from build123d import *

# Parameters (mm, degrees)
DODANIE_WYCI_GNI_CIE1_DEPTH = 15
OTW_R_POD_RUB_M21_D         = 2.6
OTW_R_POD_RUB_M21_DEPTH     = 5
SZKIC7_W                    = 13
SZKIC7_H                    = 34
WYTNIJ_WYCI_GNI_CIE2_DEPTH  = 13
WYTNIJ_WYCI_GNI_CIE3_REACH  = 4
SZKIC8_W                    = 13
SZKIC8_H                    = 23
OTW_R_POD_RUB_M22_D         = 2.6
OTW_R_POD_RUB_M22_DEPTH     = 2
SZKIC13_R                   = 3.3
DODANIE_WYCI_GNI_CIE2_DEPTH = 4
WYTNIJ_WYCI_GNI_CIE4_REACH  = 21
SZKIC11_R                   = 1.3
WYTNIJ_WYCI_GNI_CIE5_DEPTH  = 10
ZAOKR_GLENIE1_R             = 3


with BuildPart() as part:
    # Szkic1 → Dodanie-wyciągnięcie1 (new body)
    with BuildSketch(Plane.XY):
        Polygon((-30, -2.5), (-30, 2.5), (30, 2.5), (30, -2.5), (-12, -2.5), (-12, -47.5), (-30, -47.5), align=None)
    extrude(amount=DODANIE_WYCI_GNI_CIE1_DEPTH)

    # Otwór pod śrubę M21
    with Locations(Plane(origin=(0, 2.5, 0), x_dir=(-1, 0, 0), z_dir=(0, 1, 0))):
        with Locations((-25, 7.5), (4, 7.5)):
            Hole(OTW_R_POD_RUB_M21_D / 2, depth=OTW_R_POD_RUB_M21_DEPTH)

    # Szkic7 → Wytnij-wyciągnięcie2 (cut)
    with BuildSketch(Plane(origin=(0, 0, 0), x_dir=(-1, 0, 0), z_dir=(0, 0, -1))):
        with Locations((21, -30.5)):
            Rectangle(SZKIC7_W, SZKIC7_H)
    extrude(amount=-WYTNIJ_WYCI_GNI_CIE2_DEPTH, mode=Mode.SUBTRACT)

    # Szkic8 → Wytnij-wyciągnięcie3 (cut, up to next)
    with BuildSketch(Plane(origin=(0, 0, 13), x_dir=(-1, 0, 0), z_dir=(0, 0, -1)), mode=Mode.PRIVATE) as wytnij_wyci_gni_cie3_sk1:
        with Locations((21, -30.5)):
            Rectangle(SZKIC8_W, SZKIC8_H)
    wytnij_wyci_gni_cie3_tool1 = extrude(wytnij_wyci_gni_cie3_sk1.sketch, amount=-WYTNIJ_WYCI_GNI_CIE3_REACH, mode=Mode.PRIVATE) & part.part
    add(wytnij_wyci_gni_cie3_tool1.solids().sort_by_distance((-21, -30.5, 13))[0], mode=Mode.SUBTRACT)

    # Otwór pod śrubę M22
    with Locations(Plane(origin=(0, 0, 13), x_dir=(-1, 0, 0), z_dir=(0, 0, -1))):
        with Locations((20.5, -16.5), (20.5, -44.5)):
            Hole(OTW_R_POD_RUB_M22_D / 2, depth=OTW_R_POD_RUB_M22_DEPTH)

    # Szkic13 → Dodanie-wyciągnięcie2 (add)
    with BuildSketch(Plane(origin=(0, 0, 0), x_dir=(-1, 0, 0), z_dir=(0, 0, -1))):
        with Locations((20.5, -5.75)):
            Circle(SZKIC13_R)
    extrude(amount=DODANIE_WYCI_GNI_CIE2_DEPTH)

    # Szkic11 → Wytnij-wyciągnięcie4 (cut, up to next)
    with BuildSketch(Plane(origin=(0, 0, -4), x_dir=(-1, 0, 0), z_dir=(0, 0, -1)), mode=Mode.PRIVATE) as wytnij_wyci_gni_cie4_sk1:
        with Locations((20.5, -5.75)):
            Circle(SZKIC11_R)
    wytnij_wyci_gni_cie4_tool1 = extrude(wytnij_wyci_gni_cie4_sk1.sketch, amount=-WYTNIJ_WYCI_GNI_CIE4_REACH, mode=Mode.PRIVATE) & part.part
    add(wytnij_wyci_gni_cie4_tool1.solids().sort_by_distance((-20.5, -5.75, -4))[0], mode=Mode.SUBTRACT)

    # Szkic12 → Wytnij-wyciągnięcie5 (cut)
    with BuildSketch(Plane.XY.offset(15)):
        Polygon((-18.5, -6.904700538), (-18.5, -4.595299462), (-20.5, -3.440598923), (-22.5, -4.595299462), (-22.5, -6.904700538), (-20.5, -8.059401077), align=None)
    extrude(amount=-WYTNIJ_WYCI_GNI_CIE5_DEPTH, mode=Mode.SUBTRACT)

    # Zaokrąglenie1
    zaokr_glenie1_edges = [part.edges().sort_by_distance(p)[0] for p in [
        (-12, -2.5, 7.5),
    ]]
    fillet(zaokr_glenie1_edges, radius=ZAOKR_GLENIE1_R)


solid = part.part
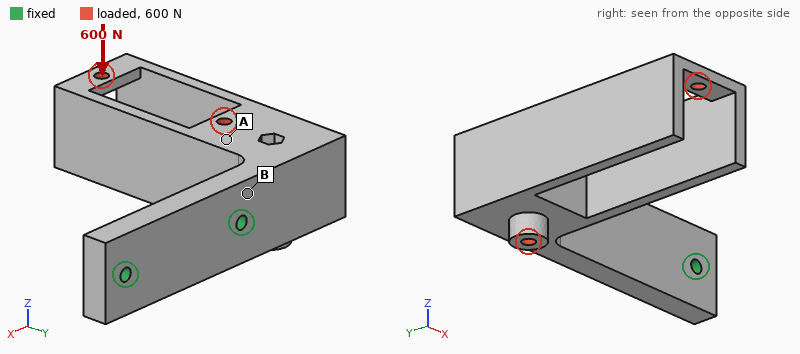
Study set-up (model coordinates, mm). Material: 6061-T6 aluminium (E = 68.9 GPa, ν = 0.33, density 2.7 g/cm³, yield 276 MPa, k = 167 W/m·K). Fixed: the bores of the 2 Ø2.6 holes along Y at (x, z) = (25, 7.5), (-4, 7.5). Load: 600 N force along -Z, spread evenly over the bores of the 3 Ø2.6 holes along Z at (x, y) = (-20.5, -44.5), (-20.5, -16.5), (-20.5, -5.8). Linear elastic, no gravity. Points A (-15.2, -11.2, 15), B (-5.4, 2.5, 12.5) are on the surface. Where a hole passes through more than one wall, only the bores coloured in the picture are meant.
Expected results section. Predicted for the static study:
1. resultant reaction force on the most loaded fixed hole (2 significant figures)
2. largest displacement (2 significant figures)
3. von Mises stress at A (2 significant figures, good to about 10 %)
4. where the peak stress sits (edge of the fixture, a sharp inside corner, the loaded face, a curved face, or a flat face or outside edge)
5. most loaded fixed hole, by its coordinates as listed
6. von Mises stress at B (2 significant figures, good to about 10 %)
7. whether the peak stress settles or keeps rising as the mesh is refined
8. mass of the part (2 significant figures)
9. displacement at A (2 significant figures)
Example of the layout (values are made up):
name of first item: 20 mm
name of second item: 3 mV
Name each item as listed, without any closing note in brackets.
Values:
resultant reaction force on the most loaded fixed hole: 870 N
largest displacement: 0.30 mm
von Mises stress at A: 12 MPa
where the peak stress sits: edge of the fixture
most loaded fixed hole, by its coordinates as listed: (-4, 7.5)
von Mises stress at B: 71 MPa
whether the peak stress settles or keeps rising as the mesh is refined: keeps rising
mass of the part: 28 g
displacement at A: 0.081 mm
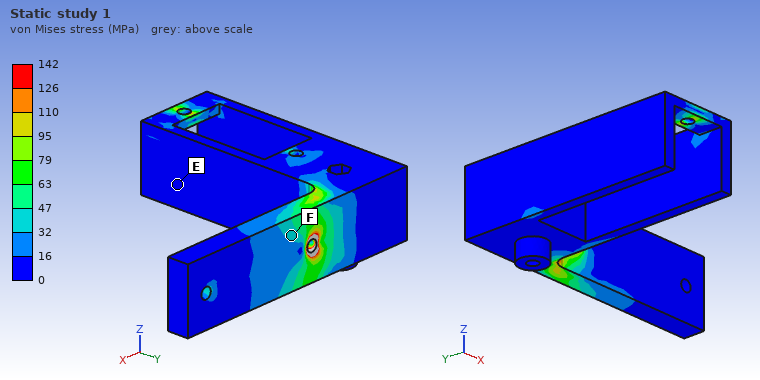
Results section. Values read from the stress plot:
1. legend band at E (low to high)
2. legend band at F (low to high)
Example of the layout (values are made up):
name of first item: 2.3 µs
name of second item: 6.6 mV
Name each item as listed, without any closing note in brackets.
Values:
legend band at E: 0 to 16 MPa
legend band at F: 32 to 47 MPa
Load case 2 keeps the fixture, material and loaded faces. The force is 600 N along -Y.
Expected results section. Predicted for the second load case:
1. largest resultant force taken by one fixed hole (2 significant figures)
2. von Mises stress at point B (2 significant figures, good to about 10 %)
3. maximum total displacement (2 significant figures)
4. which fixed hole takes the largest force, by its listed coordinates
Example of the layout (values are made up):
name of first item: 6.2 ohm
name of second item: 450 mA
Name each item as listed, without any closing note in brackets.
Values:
largest resultant force taken by one fixed hole: 680 N
von Mises stress at point B: 87 MPa
maximum total displacement: 0.36 mm
which fixed hole takes the largest force, by its listed coordinates: (-4, 7.5)
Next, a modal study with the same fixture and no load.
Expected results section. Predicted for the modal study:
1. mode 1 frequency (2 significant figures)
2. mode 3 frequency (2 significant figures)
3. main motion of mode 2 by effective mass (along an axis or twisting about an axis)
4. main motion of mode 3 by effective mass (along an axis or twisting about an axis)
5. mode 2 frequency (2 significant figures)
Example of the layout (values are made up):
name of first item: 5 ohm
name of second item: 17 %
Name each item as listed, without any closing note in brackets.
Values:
mode 1 frequency: 1300 Hz
mode 3 frequency: 4100 Hz
main motion of mode 2 by effective mass: along Z
main motion of mode 3 by effective mass: along Y
mode 2 frequency: 2000 Hz
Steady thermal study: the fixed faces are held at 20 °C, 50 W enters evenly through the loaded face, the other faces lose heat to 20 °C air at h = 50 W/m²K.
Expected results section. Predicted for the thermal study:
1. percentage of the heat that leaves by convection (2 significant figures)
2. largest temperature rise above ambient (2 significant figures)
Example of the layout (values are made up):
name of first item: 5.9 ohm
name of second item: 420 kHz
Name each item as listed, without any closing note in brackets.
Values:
percentage of the heat that leaves by convection: 22 %
largest temperature rise above ambient: 71 K
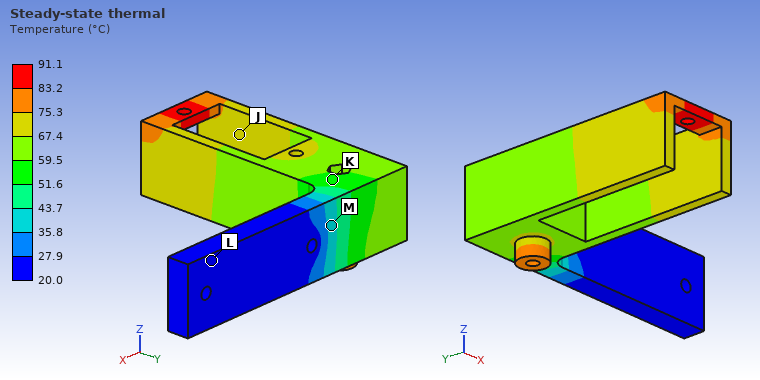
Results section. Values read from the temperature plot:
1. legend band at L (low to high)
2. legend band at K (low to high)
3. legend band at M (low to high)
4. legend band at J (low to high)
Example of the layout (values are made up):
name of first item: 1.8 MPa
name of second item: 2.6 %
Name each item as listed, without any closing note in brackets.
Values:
legend band at L: 20.0 to 27.9 °C
legend band at K: 51.6 to 59.5 °C
legend band at M: 35.8 to 43.7 °C
legend band at J: 67.4 to 75.3 °C
